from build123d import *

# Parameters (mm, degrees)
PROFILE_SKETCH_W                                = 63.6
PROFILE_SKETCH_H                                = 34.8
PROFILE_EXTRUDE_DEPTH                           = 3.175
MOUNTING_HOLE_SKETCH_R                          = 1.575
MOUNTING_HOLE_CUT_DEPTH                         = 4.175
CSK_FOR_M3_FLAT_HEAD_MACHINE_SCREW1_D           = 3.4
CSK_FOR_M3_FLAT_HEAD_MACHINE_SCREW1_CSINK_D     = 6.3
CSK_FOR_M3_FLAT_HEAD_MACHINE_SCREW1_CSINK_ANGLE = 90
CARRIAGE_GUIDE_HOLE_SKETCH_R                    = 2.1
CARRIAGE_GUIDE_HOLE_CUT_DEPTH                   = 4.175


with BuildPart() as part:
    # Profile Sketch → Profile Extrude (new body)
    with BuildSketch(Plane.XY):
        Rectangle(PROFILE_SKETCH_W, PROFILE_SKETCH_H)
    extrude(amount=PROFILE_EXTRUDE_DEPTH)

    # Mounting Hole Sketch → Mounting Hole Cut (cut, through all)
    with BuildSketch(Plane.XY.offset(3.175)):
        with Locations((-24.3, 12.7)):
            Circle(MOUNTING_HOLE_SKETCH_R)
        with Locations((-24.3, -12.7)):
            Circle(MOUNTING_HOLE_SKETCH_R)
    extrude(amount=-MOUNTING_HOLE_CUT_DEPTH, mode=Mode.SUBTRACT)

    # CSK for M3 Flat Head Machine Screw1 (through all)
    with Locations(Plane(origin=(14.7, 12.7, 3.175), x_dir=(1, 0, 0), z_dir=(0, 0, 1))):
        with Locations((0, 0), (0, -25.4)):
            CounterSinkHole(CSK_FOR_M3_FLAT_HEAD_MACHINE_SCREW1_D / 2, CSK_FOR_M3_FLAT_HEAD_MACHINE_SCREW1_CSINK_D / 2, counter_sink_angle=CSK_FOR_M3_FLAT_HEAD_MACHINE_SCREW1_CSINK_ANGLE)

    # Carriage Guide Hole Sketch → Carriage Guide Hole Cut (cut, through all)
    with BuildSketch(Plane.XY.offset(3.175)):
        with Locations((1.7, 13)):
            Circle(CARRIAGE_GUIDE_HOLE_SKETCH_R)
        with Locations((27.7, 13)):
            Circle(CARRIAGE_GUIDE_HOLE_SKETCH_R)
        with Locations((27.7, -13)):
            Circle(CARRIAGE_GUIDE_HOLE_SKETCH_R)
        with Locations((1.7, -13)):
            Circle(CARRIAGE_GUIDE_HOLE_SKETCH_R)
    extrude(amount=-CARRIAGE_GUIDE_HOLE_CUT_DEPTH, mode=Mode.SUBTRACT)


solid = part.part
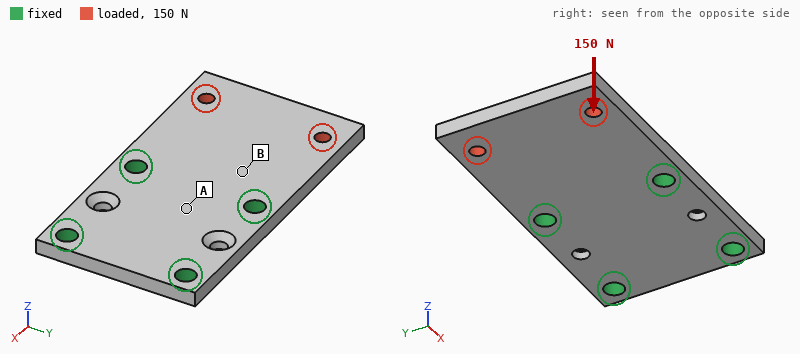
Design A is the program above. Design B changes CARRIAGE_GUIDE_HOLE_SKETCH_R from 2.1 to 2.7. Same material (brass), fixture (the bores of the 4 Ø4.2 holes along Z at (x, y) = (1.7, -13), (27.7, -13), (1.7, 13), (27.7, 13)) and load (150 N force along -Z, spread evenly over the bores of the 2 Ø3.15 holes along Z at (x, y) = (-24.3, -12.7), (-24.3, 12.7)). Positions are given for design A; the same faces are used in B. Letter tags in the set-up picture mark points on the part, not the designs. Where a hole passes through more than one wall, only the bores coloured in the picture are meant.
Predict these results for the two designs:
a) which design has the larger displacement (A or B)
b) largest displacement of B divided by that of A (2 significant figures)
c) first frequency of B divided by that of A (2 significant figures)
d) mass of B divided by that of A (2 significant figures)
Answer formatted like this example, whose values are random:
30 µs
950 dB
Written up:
A
0.92
1.0
0.98
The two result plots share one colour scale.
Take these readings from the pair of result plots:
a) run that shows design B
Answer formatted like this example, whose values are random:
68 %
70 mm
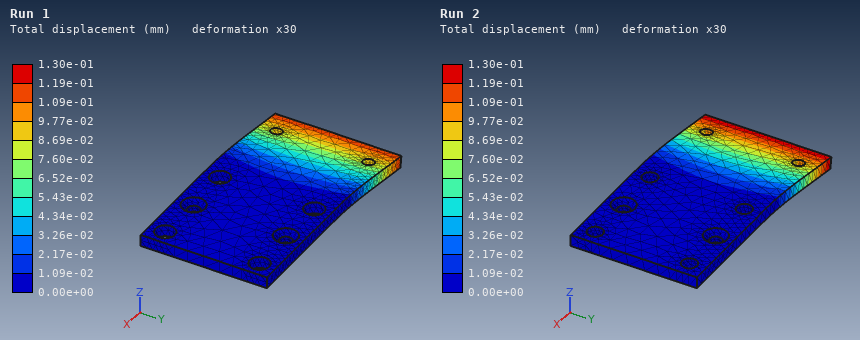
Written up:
Run 1
